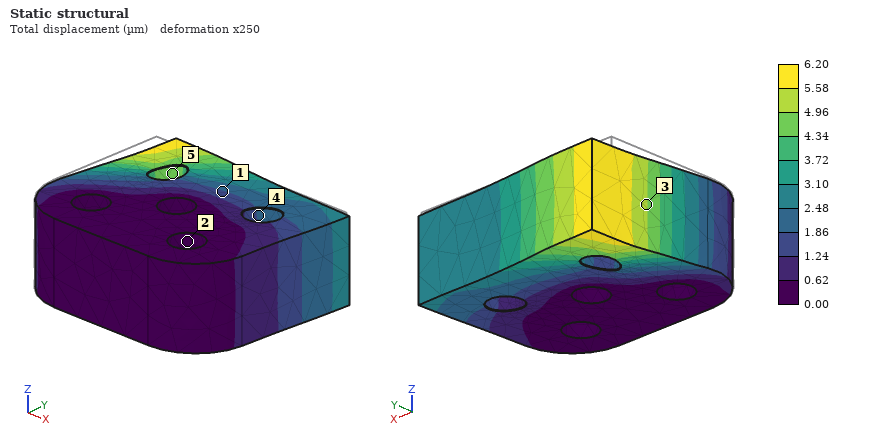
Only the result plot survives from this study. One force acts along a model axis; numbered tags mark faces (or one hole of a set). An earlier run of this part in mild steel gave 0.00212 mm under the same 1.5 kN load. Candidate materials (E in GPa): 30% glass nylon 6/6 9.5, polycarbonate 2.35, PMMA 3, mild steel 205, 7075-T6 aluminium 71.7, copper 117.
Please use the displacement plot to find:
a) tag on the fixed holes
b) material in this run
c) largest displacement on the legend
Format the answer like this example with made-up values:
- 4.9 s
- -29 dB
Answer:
- 2
- 7075-T6 aluminium
- 6.20 µm
